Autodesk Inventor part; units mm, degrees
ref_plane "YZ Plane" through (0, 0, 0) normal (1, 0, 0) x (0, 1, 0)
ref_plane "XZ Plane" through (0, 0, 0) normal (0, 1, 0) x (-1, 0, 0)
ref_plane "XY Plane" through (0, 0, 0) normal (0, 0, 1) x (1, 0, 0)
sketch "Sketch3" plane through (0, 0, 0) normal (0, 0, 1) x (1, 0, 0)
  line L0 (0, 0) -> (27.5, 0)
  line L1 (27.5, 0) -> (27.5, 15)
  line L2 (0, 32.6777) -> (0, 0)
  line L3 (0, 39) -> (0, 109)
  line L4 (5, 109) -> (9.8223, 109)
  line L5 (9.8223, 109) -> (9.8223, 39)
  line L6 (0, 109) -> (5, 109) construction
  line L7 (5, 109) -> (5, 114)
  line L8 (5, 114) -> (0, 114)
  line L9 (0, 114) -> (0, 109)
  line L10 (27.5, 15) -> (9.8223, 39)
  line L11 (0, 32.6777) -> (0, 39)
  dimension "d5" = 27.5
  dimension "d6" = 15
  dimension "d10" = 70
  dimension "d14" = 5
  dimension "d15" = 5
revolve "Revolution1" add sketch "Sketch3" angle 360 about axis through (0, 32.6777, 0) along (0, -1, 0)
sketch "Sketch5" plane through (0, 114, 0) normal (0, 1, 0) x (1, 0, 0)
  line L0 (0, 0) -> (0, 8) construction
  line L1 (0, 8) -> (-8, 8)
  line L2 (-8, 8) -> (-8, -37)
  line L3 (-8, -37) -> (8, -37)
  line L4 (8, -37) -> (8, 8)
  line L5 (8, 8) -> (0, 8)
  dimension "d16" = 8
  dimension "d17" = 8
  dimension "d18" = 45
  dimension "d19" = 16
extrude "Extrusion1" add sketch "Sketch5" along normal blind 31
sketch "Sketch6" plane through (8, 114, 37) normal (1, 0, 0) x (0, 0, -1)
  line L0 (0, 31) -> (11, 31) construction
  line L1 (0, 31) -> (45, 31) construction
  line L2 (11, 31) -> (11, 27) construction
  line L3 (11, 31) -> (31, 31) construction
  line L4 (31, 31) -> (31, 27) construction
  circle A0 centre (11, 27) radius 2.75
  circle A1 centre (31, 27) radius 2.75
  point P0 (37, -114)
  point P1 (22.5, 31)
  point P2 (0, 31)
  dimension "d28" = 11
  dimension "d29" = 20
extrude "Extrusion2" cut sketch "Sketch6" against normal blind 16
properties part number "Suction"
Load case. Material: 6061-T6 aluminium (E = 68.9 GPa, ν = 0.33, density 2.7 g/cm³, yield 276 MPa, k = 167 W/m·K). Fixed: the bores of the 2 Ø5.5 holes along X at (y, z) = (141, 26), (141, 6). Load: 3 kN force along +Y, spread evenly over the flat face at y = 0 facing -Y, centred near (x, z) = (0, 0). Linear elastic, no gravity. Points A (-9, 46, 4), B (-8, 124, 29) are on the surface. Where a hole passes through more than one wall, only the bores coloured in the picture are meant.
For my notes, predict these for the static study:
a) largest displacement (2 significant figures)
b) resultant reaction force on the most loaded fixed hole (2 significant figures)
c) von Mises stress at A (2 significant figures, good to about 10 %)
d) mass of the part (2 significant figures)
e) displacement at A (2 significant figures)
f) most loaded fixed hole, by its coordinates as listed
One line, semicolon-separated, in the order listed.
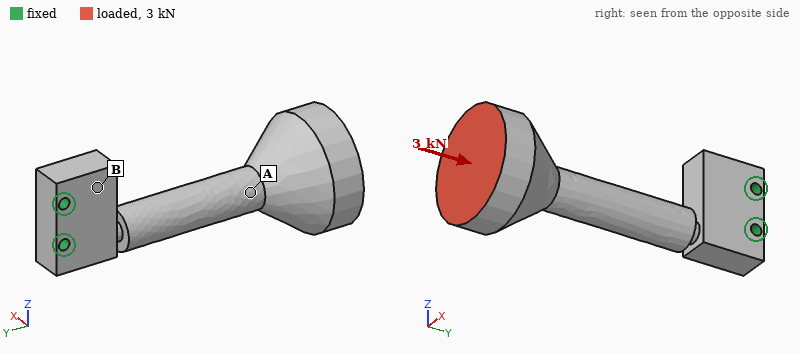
46 µm; 3.5 kN; 9.7 MPa; 290 g; 29 µm; (141, 6)
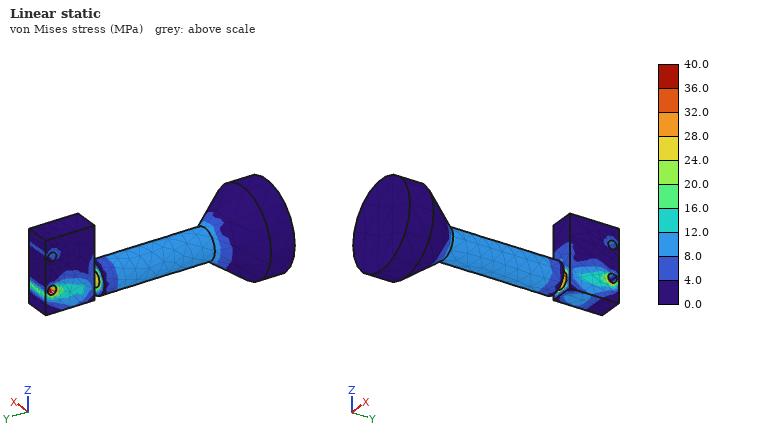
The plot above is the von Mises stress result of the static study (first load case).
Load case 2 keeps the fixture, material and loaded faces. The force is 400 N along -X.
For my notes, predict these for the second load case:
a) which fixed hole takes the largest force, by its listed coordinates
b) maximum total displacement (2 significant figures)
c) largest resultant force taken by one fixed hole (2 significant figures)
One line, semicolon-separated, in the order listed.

(141, 6); 1.9 mm; 250 N
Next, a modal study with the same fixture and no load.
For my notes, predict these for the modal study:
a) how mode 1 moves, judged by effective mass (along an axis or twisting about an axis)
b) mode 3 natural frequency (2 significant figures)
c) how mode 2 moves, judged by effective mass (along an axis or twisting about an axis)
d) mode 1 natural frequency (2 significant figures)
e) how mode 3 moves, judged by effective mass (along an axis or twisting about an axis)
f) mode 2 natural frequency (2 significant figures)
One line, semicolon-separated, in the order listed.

along X; 920 Hz; along Z; 200 Hz; twisting about Y; 210 Hz
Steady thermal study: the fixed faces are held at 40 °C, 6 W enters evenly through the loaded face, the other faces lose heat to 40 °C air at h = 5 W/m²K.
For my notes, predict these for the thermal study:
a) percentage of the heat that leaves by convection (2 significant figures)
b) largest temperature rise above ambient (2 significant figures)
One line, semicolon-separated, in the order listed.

11 %; 14 K
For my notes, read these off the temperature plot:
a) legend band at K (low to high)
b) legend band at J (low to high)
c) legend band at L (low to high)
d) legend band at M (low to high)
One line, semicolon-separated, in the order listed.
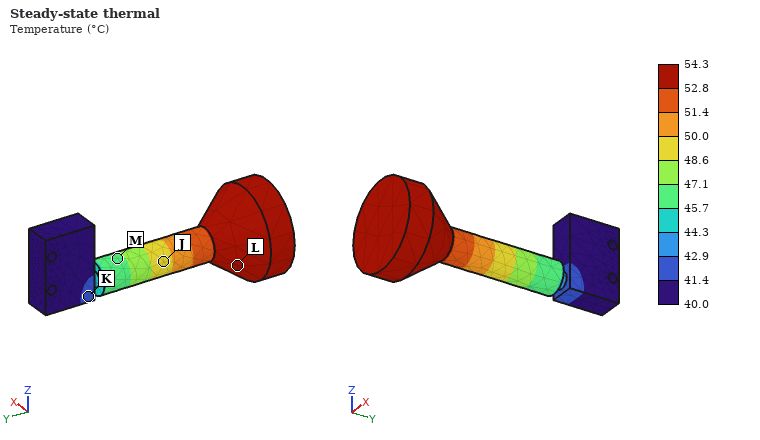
41.4 to 42.9 °C; 48.6 to 50.0 °C; 52.8 to 54.3 °C; 45.7 to 47.1 °C
